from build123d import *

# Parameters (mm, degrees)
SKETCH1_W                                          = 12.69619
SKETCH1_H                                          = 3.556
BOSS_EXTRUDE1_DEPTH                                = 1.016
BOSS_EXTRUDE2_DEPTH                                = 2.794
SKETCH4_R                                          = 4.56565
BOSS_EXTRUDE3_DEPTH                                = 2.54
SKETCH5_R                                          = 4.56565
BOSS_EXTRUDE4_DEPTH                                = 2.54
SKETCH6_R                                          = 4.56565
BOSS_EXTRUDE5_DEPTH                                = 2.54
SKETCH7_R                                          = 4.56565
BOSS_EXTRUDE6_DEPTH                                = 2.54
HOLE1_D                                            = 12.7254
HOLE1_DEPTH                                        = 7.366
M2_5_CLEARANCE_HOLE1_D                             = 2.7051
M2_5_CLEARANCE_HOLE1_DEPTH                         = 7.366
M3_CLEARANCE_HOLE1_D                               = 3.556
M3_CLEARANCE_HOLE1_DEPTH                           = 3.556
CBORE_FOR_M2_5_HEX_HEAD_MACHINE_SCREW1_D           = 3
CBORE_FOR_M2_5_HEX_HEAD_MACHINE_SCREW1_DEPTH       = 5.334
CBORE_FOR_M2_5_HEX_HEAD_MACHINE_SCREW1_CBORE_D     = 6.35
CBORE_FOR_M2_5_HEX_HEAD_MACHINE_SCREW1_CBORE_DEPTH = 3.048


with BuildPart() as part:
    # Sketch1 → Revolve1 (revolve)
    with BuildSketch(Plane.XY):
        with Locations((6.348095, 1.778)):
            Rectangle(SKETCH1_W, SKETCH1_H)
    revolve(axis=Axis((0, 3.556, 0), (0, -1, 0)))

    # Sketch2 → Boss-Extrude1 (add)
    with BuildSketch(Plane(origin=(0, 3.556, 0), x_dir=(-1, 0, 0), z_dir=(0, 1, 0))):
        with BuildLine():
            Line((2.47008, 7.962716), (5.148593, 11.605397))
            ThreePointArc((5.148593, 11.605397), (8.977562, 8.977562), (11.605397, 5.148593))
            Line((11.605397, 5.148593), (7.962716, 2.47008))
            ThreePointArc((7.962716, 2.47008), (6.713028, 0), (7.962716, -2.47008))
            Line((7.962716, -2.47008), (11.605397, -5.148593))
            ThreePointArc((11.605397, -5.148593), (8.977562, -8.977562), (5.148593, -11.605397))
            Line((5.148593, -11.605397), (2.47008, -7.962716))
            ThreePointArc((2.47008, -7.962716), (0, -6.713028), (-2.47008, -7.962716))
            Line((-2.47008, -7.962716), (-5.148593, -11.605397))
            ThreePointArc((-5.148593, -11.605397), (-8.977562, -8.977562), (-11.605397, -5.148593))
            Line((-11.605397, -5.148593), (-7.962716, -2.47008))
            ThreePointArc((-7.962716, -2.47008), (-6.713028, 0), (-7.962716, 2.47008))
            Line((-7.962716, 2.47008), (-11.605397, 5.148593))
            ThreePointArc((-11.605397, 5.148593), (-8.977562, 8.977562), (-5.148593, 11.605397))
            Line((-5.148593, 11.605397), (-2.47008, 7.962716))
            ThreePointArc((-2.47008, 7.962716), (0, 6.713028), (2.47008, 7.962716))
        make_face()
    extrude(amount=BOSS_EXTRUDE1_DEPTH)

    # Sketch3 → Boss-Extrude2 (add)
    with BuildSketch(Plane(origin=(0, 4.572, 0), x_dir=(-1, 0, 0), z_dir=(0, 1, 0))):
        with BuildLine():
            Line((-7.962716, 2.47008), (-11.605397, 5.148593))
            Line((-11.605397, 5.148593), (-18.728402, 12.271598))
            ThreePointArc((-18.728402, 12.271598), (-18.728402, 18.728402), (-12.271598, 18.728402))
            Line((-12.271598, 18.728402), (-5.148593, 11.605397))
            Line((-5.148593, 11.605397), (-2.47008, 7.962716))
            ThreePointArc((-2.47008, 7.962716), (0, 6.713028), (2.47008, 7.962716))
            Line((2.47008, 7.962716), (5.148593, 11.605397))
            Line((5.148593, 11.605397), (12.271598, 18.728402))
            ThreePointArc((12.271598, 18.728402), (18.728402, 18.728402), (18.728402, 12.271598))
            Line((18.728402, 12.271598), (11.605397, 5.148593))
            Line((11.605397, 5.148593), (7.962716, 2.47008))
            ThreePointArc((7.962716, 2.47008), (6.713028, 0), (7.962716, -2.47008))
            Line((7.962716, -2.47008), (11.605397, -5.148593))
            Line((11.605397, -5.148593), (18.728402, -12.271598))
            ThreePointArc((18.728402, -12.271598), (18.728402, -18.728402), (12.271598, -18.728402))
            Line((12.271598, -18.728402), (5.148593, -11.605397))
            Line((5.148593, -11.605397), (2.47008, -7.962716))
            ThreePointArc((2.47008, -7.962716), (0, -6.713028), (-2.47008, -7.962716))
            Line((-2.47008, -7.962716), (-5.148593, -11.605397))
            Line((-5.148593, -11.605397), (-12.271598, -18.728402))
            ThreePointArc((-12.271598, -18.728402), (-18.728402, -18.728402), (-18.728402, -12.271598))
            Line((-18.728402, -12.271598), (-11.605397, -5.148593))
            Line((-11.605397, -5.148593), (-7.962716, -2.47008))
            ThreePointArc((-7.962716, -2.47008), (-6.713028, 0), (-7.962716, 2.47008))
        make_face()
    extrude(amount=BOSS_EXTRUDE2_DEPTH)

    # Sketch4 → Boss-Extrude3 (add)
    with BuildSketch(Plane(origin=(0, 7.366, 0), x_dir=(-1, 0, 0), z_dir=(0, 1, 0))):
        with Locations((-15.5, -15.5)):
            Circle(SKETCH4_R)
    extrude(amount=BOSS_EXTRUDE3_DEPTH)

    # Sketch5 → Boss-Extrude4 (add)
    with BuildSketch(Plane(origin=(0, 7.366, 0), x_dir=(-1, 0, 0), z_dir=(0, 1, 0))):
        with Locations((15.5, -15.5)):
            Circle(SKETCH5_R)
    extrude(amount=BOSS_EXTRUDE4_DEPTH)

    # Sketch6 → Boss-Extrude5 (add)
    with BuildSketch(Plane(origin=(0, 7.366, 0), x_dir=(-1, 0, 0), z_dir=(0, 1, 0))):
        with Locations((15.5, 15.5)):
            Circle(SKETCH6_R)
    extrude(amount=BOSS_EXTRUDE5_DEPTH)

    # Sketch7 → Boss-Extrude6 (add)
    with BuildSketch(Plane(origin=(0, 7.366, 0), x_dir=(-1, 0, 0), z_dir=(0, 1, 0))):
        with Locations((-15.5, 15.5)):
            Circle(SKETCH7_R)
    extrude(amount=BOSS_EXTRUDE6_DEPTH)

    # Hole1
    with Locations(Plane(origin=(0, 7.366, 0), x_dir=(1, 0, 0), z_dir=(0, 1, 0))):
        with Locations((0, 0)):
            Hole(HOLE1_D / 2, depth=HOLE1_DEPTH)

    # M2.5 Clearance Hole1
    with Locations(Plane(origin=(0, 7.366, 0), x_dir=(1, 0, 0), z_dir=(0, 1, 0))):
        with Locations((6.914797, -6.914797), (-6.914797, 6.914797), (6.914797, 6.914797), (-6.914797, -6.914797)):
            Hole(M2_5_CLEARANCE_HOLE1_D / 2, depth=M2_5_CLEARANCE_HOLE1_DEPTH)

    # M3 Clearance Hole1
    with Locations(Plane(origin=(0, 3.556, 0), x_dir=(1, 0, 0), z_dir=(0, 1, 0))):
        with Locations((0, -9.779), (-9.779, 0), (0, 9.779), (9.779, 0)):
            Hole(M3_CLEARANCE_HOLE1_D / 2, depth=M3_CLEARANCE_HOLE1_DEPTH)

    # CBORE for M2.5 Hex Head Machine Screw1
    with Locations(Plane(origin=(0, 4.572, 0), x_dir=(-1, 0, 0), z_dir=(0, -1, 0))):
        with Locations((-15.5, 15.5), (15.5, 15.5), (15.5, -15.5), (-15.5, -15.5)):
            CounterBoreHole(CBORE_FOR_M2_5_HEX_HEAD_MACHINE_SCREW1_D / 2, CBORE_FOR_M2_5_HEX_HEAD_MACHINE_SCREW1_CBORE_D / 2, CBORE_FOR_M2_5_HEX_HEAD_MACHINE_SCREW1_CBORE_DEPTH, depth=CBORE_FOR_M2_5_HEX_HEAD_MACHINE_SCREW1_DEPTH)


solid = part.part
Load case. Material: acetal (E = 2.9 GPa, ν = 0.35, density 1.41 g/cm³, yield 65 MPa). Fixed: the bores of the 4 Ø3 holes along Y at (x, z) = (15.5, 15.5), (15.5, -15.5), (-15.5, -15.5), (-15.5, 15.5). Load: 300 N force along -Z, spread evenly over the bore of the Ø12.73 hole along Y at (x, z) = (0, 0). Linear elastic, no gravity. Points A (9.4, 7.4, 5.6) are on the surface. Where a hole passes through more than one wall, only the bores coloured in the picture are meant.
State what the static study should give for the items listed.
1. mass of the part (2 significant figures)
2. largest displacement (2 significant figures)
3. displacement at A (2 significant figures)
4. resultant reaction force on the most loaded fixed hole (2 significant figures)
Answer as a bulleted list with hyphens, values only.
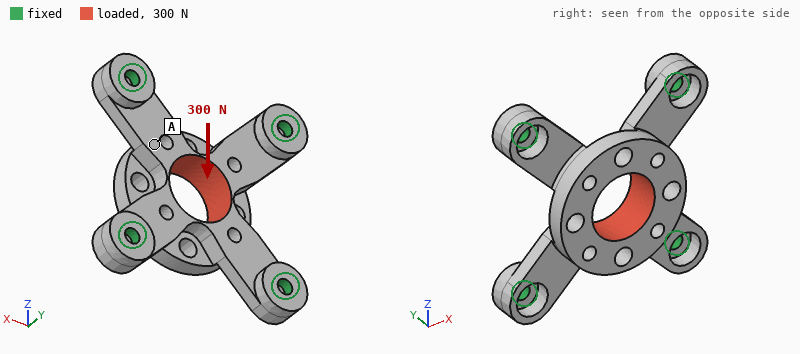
- 4.8 g
- 77 µm
- 45 µm
- 91 N
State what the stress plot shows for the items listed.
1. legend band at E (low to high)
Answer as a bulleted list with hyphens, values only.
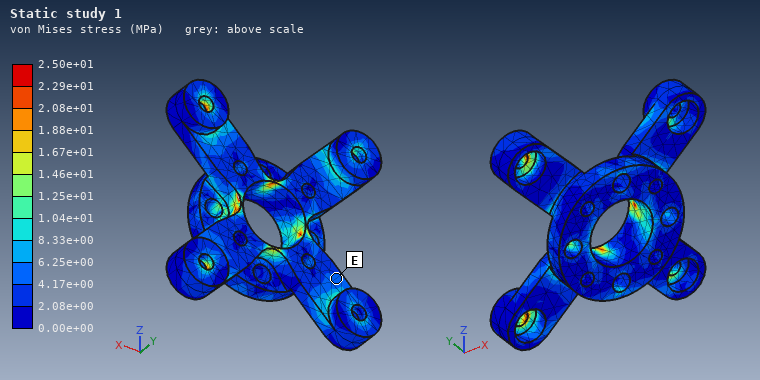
- 4.17e+00 to 6.25e+00 MPa
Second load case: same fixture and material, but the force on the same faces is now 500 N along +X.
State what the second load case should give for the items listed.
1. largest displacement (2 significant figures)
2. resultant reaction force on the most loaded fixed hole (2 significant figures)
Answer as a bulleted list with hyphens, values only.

- 0.13 mm
- 150 N
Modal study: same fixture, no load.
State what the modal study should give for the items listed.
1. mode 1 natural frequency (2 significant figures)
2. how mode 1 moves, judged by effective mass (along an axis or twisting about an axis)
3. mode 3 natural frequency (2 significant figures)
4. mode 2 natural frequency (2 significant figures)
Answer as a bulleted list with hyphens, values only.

- 4200 Hz
- along Y
- 5400 Hz
- 5400 Hz
